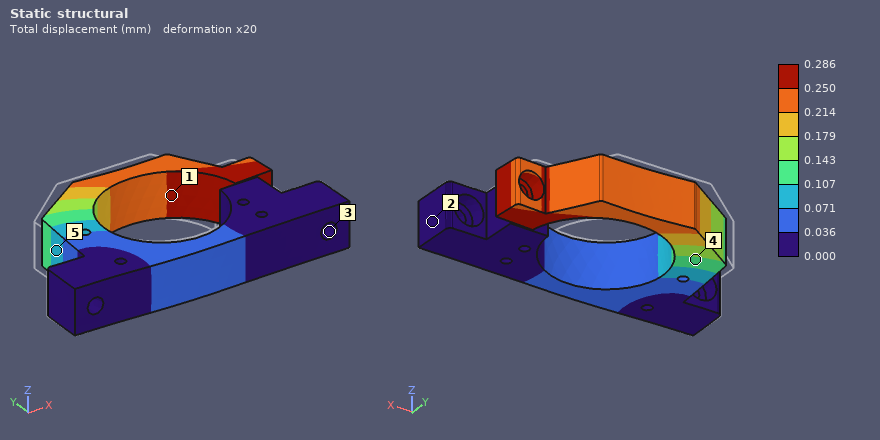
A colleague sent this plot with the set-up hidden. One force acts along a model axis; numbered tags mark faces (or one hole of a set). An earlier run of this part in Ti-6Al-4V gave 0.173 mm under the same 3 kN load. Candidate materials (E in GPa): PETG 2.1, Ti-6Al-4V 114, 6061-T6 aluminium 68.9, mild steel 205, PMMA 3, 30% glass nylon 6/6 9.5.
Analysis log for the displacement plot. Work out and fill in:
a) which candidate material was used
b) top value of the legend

6061-T6 aluminium
0.286 mm
